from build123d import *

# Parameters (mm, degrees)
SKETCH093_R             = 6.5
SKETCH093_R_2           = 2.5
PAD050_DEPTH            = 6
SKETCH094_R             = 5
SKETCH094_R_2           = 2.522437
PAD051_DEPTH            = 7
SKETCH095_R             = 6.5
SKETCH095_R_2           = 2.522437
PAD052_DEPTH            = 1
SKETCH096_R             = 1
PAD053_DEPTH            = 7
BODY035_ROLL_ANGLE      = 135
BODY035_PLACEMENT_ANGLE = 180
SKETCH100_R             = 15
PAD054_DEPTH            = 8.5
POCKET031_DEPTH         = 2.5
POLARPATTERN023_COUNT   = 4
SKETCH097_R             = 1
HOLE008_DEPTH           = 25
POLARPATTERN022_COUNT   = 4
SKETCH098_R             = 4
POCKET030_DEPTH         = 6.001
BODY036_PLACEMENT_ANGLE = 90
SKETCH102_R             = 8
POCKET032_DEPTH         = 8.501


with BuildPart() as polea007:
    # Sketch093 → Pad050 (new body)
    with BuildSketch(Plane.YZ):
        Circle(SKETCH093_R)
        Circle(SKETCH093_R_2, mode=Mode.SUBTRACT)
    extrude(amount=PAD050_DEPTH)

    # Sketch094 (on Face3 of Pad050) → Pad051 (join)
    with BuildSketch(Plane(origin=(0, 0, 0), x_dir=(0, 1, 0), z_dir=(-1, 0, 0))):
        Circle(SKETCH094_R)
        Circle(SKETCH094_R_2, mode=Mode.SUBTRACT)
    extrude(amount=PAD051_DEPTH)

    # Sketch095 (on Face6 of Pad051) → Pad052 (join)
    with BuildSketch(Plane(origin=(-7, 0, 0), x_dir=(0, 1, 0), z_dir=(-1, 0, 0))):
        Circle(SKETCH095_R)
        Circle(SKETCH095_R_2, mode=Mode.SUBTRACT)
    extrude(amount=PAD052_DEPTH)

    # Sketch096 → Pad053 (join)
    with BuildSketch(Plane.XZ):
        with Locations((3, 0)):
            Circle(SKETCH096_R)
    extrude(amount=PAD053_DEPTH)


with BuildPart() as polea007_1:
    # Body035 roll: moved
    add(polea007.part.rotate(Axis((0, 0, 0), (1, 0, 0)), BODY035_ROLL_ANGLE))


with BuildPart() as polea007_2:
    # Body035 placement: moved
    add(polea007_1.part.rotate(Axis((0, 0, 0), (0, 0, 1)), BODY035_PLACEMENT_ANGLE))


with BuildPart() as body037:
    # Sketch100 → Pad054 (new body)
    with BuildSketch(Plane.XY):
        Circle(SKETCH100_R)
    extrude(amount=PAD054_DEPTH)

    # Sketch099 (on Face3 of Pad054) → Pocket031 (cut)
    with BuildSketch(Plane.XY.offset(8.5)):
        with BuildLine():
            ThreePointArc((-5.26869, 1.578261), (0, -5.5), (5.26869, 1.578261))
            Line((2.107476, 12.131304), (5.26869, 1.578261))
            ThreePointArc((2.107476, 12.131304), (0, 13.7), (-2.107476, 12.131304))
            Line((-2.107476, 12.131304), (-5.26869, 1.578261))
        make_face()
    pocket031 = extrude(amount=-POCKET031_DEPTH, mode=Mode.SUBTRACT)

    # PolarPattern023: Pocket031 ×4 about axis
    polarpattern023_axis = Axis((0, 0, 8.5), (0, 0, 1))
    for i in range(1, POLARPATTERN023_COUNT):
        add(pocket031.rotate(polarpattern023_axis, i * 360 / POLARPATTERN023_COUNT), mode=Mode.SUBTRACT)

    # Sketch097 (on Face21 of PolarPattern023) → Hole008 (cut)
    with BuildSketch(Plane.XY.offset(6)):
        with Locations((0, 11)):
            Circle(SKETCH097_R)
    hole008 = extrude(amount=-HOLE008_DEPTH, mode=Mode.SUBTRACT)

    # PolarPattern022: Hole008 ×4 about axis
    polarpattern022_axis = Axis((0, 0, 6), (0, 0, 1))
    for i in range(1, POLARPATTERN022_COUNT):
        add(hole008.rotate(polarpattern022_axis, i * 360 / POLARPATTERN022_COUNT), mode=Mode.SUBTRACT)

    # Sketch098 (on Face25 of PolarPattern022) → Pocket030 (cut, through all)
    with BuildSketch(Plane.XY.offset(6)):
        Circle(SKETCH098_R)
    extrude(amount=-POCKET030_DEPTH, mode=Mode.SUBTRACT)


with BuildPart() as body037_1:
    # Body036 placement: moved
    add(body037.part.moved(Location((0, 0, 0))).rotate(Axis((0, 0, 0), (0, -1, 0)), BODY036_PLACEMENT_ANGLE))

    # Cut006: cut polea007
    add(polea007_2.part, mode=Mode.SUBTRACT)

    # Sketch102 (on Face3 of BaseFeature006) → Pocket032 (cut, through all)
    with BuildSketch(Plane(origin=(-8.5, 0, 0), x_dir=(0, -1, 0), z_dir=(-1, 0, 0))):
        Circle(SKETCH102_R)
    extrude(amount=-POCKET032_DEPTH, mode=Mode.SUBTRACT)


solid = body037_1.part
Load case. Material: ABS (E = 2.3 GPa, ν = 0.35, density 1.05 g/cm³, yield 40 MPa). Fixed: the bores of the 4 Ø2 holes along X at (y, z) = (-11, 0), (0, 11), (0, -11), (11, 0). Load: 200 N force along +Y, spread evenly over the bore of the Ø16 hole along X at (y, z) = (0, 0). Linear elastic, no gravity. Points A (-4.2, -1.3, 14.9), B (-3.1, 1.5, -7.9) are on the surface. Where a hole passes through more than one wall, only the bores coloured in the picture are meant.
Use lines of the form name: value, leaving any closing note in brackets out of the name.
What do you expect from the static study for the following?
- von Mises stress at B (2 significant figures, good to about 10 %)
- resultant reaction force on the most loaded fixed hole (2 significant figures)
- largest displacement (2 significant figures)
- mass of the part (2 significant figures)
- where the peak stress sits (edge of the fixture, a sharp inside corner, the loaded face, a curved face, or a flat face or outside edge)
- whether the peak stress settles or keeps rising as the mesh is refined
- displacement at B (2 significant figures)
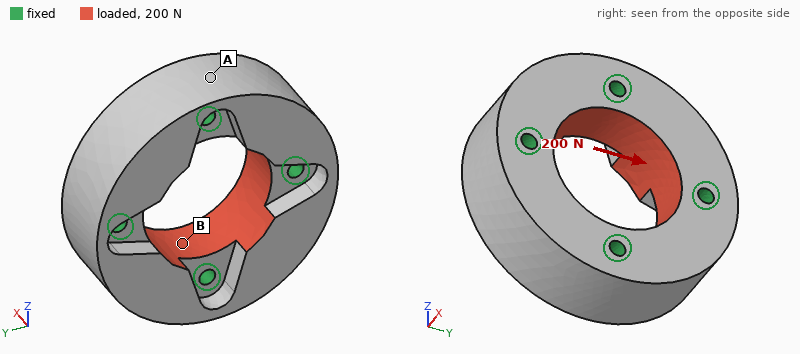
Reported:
von Mises stress at B: 1.0 MPa
resultant reaction force on the most loaded fixed hole: 56 N
largest displacement: 4.9 µm
mass of the part: 4.1 g
where the peak stress sits: edge of the fixture
whether the peak stress settles or keeps rising as the mesh is refined: keeps rising
displacement at B: 2.9 µm
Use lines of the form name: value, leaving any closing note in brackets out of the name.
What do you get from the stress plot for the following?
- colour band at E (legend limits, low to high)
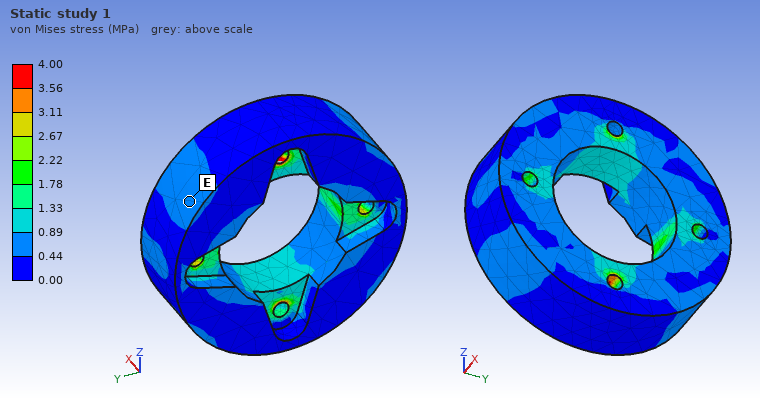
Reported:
colour band at E: 0.44 to 0.89 MPa
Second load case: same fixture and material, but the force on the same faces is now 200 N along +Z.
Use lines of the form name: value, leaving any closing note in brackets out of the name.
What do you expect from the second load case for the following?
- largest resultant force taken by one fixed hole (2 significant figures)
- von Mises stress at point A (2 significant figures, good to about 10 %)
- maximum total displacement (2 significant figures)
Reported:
largest resultant force taken by one fixed hole: 56 N
von Mises stress at point A: 0.59 MPa
maximum total displacement: 4.9 µm
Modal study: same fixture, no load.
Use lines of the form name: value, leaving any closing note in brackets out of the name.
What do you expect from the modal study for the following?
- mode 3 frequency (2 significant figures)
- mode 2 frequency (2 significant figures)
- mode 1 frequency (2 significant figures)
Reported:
mode 3 frequency: 13 kHz
mode 2 frequency: 13 kHz
mode 1 frequency: 12 kHz
